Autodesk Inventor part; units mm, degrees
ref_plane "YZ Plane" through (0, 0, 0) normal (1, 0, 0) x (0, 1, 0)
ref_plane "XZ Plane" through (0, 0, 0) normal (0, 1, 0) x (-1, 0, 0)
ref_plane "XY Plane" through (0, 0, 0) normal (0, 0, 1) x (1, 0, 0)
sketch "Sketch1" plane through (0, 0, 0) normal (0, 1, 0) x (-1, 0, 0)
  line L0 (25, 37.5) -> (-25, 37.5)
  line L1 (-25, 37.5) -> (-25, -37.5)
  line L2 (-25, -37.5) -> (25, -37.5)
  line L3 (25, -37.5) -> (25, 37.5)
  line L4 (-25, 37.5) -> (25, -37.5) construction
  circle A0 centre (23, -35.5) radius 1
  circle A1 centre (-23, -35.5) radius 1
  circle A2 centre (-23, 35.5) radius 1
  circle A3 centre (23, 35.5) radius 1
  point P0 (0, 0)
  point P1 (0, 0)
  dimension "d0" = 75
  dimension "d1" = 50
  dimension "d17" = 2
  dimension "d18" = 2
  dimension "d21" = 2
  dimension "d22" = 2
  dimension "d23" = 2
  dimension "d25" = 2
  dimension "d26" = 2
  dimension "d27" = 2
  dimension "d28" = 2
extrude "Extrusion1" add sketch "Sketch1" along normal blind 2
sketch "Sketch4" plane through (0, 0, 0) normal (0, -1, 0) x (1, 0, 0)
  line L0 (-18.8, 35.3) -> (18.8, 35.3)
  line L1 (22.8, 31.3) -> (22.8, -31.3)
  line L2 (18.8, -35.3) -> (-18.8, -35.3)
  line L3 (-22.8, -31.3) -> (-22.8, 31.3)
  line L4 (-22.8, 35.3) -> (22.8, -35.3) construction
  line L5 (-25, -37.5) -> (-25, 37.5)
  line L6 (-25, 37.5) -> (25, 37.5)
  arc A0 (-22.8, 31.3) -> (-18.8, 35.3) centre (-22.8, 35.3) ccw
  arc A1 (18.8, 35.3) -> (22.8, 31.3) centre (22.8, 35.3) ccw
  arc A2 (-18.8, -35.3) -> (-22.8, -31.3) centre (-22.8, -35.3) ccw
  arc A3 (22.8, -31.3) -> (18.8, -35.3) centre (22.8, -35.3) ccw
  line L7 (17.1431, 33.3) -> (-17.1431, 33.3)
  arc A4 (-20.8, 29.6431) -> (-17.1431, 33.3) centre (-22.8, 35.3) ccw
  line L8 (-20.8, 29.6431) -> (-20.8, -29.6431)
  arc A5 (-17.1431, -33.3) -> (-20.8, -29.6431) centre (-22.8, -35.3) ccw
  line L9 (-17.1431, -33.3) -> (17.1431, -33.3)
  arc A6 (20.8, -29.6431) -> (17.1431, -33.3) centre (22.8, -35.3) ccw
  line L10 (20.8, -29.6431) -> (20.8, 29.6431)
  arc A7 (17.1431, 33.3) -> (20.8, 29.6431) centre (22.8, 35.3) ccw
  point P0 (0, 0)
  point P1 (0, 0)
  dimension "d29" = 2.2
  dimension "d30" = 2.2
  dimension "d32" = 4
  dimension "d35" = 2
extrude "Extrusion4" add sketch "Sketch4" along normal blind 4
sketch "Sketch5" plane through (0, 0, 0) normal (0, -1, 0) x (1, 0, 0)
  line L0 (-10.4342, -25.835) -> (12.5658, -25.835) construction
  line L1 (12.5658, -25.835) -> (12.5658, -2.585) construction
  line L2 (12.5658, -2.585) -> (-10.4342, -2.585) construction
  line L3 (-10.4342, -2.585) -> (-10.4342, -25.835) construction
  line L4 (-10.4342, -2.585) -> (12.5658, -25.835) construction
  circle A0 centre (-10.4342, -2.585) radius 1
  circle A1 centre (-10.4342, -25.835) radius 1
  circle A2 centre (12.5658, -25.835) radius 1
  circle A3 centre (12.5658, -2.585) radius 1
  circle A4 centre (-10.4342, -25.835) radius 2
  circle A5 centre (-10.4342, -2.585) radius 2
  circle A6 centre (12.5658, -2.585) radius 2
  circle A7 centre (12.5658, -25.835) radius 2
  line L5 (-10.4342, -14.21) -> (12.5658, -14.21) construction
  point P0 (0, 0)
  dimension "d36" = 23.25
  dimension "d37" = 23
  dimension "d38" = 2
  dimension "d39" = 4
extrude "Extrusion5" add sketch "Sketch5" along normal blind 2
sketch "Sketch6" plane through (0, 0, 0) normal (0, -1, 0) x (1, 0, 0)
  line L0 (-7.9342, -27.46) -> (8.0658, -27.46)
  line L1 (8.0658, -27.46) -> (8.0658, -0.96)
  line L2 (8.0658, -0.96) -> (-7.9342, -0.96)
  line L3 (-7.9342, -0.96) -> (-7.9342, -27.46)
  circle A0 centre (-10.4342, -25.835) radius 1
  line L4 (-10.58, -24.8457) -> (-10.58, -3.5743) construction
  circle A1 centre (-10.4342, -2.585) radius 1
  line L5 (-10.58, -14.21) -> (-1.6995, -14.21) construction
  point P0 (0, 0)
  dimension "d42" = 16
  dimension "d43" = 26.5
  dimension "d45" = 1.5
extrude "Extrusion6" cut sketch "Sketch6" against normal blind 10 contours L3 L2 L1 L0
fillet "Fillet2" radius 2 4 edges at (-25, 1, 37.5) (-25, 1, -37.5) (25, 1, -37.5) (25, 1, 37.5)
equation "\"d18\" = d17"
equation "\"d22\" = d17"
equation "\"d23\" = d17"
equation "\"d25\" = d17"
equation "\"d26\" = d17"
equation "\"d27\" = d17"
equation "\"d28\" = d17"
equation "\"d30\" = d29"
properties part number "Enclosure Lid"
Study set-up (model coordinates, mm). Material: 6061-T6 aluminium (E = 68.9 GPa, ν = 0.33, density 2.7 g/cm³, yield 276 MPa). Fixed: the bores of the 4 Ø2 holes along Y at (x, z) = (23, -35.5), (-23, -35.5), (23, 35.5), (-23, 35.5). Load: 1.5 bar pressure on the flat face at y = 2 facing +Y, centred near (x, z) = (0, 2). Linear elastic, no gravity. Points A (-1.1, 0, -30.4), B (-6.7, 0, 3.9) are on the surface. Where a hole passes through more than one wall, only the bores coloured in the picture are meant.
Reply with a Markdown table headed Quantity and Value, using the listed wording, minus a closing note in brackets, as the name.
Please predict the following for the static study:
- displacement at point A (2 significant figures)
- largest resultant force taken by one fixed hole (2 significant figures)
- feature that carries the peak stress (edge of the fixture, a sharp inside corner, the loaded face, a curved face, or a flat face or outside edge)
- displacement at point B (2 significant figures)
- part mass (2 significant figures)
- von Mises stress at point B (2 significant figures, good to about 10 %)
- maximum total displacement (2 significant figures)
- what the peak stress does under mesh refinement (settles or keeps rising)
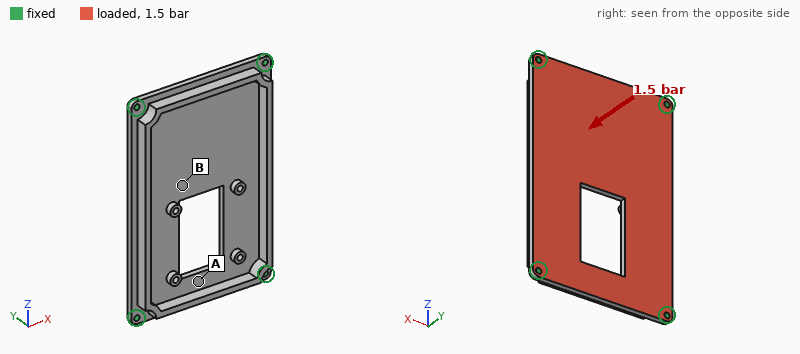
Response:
| Quantity | Value |
|---|---|
| displacement at point A | 0.048 mm |
| largest resultant force taken by one fixed hole | 200 N |
| feature that carries the peak stress | edge of the fixture |
| displacement at point B | 0.16 mm |
| part mass | 23 g |
| von Mises stress at point B | 26 MPa |
| maximum total displacement | 0.19 mm |
| what the peak stress does under mesh refinement | keeps rising |
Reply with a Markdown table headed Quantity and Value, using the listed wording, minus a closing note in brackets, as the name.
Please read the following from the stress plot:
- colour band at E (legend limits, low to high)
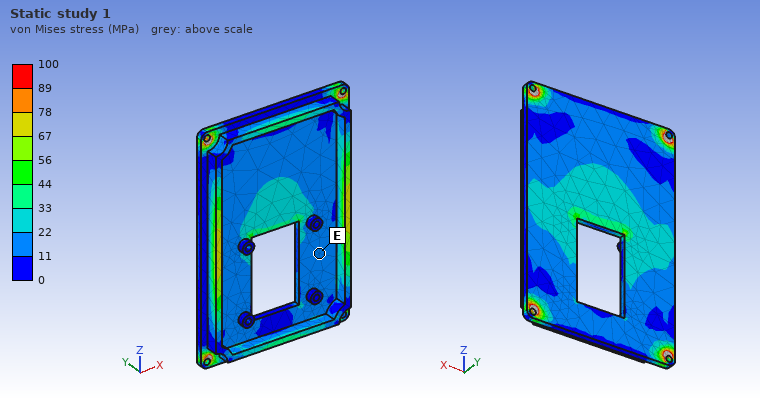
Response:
| Quantity | Value |
|---|---|
| colour band at E | 11 to 22 MPa |
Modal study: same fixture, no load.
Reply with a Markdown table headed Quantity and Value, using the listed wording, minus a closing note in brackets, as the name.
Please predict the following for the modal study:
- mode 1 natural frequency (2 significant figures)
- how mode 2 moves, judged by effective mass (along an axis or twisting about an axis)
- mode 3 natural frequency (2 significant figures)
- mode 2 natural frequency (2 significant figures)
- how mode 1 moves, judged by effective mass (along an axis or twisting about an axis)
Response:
| Quantity | Value |
|---|---|
| mode 1 natural frequency | 2400 Hz |
| how mode 2 moves, judged by effective mass | twisting about Z |
| mode 3 natural frequency | 5600 Hz |
| mode 2 natural frequency | 3600 Hz |
| how mode 1 moves, judged by effective mass | along Y |
